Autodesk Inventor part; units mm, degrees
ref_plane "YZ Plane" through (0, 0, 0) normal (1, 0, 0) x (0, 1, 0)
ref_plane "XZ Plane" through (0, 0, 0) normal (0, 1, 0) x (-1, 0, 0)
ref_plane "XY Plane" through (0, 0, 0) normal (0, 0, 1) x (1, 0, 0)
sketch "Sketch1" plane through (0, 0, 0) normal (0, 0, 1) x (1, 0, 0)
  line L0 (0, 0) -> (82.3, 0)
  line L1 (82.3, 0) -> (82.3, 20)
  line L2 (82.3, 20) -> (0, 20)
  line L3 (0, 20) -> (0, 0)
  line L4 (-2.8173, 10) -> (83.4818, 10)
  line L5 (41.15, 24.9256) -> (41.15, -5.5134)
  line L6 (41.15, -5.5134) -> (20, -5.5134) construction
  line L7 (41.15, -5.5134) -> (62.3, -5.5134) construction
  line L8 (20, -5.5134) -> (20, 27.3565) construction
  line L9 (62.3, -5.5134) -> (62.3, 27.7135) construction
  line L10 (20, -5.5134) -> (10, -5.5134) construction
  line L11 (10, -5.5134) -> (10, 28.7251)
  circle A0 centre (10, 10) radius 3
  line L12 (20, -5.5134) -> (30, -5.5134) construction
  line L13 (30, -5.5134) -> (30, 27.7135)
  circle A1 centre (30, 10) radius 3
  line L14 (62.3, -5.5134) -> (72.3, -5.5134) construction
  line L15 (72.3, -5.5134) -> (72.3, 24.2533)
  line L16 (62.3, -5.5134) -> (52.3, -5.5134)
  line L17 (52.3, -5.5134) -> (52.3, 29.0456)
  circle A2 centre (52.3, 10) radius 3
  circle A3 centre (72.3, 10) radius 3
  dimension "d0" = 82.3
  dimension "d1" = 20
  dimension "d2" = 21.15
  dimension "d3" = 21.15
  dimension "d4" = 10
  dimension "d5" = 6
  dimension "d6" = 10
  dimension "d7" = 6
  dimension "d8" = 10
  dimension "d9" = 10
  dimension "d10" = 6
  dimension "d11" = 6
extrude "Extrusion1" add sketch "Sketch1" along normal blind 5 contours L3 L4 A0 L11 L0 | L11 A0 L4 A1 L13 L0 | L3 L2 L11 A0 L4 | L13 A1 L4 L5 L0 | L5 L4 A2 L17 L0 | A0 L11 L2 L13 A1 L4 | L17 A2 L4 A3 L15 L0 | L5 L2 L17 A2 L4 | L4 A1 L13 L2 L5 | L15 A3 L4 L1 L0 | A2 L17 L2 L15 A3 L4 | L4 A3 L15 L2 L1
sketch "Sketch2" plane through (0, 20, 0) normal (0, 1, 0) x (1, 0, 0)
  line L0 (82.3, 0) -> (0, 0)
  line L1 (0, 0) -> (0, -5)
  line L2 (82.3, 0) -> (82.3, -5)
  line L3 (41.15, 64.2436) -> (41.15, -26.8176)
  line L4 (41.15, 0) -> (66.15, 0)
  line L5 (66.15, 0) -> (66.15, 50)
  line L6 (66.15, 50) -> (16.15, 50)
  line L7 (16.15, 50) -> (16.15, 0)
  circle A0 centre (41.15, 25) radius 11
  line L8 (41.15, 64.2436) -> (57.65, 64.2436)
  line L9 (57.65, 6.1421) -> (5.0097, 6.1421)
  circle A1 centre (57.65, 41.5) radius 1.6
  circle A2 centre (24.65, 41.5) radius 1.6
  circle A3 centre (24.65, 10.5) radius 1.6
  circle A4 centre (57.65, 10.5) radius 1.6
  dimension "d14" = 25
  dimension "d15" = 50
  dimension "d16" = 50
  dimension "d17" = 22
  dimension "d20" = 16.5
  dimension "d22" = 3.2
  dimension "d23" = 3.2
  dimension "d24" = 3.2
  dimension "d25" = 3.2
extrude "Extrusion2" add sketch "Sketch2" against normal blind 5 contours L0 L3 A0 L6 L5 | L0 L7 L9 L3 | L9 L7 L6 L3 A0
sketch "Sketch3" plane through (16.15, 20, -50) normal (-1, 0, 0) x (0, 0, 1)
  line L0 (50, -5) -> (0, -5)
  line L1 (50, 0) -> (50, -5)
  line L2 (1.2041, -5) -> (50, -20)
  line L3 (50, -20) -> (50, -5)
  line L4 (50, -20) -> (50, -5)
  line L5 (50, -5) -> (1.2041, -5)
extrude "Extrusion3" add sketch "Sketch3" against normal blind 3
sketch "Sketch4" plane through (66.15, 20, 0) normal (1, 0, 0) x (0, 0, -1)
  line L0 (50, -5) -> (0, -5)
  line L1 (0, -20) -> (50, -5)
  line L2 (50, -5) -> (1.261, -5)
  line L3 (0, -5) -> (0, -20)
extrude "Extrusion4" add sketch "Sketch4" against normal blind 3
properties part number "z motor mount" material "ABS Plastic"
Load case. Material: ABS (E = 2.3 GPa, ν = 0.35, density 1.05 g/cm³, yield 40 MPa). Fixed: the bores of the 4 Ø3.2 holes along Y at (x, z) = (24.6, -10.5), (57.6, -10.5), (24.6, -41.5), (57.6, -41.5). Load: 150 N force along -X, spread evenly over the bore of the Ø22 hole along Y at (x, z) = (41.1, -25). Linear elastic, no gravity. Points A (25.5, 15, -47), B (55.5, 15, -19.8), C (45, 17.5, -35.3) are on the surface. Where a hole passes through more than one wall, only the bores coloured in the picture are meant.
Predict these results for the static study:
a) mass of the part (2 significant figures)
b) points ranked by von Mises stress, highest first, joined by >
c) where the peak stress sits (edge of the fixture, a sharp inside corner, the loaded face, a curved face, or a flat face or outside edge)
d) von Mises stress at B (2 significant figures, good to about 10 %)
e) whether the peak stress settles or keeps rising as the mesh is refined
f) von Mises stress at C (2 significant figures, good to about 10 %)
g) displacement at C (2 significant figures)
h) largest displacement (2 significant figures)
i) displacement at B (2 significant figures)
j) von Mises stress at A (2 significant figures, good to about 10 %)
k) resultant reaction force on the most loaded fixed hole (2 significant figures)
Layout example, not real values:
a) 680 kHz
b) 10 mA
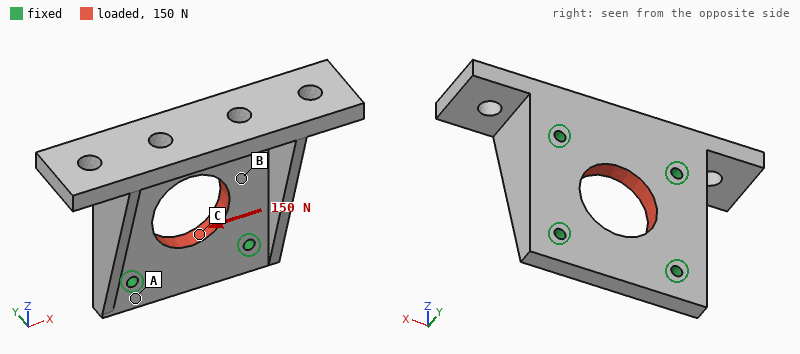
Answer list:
a) 21 g
b) C > B > A
c) edge of the fixture
d) 0.45 MPa
e) keeps rising
f) 0.78 MPa
g) 3.9 µm
h) 6.1 µm
i) 4.4 µm
j) 0.17 MPa
k) 40 N
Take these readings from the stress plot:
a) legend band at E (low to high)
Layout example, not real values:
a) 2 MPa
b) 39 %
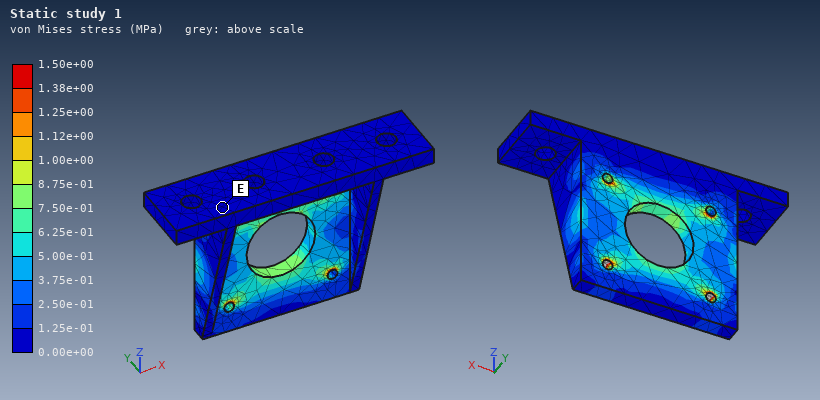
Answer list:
a) 0.00e+00 to 1.25e-01 MPa
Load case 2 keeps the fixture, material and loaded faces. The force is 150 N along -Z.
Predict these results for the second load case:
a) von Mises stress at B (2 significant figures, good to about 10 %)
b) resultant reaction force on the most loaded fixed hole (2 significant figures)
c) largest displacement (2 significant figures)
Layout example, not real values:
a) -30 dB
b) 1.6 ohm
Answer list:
a) 0.60 MPa
b) 39 N
c) 7.0 µm
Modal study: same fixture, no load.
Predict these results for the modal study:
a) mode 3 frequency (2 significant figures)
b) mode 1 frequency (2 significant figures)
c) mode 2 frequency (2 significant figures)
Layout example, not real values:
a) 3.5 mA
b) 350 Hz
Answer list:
a) 2500 Hz
b) 1800 Hz
c) 2100 Hz
